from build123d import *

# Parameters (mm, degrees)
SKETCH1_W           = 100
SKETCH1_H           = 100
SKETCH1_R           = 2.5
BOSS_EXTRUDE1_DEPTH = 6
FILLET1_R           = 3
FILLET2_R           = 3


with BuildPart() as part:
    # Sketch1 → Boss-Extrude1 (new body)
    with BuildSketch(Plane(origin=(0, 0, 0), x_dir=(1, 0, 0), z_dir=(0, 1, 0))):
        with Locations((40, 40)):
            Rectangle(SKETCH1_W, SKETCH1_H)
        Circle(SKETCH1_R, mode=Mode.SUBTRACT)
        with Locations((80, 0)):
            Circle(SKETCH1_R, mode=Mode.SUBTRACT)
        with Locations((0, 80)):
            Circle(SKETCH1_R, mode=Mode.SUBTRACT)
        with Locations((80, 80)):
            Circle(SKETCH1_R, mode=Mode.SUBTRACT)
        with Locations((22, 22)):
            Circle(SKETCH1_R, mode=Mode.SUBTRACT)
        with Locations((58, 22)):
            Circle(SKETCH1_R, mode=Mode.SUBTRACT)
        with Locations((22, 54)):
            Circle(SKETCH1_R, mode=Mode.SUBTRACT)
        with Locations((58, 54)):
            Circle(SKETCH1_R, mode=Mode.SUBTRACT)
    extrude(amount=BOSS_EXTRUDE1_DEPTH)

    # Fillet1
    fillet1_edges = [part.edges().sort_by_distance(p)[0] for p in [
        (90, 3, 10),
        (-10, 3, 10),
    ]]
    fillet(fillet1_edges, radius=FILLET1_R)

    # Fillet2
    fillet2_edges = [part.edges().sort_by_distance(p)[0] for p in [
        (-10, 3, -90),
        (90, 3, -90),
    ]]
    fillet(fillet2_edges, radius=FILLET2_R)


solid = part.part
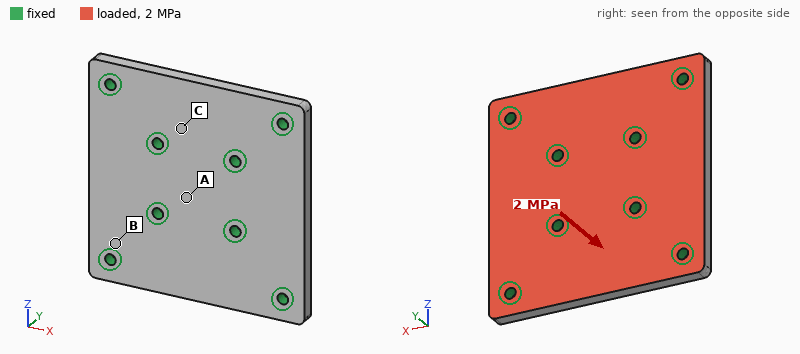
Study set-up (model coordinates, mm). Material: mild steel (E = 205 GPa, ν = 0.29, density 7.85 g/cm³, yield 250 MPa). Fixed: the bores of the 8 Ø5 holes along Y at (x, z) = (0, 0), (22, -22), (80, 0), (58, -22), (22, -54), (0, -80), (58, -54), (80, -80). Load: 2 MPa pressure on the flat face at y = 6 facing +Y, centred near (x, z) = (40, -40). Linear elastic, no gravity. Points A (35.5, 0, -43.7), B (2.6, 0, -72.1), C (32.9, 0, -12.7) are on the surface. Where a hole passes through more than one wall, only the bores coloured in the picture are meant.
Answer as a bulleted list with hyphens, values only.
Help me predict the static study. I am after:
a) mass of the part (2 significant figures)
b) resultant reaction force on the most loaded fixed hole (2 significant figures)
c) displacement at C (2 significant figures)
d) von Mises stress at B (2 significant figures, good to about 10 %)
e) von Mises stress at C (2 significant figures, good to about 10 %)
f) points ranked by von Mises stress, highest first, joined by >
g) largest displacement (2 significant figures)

- 460 g
- 3.0 kN
- 8.4 µm
- 50 MPa
- 25 MPa
- B > C > A
- 37 µm
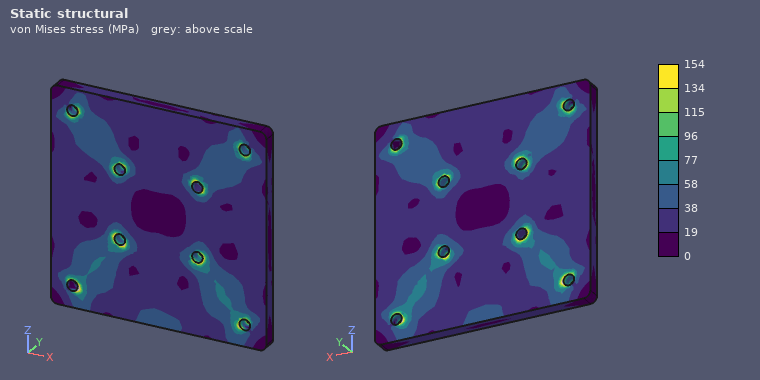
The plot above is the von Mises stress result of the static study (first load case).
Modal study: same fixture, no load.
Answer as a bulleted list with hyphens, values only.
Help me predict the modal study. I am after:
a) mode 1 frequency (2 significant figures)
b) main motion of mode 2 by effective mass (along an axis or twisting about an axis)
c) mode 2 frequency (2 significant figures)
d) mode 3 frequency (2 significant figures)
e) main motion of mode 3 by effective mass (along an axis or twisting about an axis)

- 6600 Hz
- twisting about X
- 7200 Hz
- 7600 Hz
- twisting about Z
